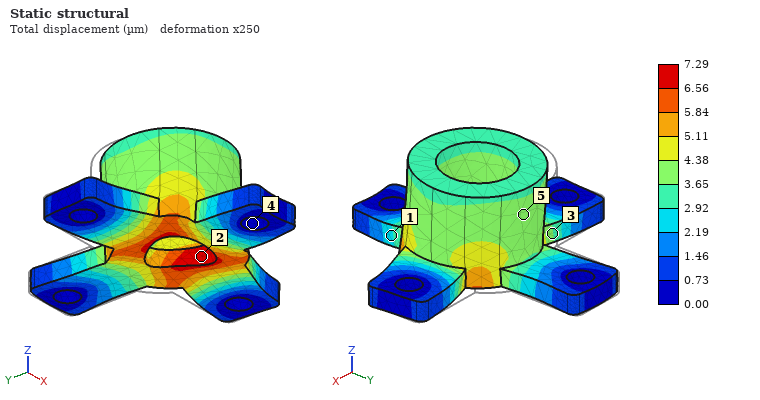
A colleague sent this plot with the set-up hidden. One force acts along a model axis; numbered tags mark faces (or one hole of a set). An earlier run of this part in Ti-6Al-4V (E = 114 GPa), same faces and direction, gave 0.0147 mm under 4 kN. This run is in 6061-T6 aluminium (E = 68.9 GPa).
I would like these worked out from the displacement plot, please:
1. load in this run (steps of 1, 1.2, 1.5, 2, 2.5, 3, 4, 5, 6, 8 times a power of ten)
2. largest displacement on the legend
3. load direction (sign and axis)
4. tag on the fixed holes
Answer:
1.2 kN
7.29 µm
-Y
4
